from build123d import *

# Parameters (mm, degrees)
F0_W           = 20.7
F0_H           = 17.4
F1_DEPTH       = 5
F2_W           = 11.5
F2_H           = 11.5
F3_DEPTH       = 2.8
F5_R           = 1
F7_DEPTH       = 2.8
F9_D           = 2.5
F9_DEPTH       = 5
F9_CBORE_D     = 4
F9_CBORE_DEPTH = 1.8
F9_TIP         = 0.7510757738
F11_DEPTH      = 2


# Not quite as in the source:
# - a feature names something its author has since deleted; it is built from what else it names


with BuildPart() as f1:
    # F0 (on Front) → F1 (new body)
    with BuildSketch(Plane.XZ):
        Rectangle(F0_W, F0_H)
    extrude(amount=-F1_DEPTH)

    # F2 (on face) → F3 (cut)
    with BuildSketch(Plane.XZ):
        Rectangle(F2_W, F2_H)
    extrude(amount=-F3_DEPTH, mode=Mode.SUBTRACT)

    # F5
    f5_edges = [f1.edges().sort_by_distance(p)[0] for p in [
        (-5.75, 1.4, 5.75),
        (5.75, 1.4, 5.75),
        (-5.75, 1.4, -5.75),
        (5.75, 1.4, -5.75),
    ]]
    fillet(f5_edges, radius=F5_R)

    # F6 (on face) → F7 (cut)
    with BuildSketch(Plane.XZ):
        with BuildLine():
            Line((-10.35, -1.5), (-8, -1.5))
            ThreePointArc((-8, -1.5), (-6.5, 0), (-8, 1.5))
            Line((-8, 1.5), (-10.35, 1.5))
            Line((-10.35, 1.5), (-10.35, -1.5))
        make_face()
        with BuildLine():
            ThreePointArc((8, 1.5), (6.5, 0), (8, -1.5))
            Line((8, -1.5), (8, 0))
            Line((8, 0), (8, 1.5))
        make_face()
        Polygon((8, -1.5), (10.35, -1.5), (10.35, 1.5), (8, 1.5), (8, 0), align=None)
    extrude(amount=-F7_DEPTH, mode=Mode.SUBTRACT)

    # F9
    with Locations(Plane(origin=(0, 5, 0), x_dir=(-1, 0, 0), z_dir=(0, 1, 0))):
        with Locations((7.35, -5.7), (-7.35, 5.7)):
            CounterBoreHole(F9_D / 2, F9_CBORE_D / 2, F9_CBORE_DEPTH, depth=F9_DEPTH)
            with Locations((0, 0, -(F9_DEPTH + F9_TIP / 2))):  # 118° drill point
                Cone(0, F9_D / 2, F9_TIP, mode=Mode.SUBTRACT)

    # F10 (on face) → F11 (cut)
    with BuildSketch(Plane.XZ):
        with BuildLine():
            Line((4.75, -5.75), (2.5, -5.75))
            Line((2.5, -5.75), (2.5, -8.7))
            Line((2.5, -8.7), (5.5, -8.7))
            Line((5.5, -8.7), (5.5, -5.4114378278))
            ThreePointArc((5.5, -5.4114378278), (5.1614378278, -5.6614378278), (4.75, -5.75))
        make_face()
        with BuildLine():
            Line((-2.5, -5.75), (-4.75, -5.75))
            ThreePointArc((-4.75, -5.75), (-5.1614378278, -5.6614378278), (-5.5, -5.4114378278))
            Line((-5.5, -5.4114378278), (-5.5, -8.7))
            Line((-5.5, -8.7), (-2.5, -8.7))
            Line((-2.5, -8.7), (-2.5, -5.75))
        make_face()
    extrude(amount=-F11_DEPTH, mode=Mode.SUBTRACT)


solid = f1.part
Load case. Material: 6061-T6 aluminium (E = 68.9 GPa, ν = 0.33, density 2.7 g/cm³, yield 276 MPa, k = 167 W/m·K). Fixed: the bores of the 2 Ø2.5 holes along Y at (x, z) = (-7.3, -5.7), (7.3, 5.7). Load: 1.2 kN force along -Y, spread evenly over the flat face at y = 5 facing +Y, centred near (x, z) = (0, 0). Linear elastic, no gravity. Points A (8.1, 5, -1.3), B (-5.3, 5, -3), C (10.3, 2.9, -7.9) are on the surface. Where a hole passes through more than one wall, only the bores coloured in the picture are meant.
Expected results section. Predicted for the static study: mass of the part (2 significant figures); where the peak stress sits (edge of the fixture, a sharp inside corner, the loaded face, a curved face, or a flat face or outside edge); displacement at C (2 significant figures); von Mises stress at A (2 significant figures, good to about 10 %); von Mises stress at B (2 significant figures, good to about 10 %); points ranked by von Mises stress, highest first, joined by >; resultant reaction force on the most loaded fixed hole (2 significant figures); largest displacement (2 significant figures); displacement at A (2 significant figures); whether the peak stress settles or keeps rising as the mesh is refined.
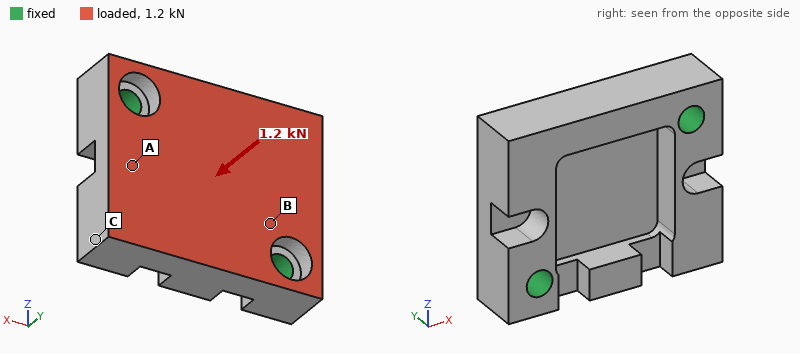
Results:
3.4 g
edge of the fixture
47 µm
38 MPa
73 MPa
B > A > C
810 N
51 µm
21 µm
keeps rising
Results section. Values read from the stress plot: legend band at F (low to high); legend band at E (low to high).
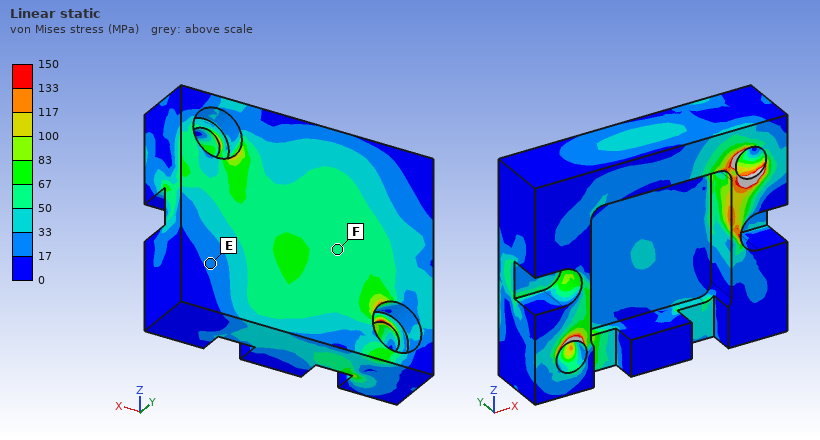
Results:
50 to 67 MPa
17 to 33 MPa
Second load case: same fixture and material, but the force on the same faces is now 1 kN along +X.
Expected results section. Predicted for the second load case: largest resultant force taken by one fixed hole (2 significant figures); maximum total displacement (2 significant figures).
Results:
530 N
22 µm
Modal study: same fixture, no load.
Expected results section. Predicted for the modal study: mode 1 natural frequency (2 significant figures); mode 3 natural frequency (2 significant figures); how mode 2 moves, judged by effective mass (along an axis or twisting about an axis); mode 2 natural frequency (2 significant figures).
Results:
14 kHz
37 kHz
along Y
19 kHz
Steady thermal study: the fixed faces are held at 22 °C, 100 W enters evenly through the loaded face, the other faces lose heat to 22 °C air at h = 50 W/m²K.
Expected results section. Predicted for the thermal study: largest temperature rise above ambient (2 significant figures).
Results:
66 K
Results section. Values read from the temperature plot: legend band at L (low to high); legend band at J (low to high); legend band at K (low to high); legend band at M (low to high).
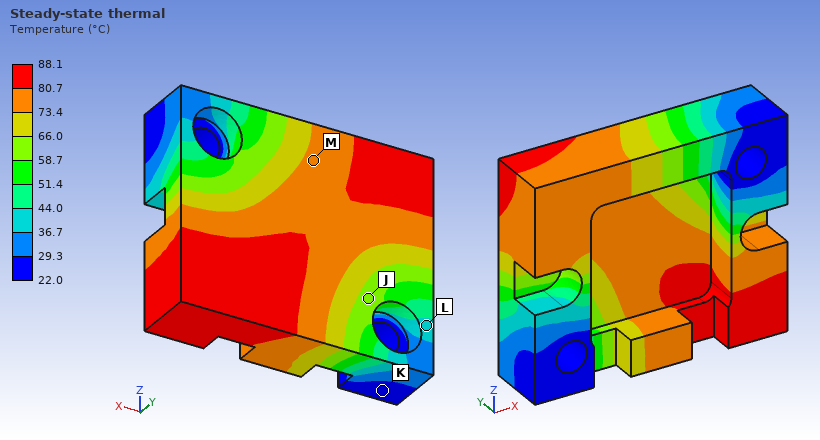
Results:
36.7 to 44.0 °C
58.7 to 66.0 °C
22.0 to 29.3 °C
73.4 to 80.7 °C
